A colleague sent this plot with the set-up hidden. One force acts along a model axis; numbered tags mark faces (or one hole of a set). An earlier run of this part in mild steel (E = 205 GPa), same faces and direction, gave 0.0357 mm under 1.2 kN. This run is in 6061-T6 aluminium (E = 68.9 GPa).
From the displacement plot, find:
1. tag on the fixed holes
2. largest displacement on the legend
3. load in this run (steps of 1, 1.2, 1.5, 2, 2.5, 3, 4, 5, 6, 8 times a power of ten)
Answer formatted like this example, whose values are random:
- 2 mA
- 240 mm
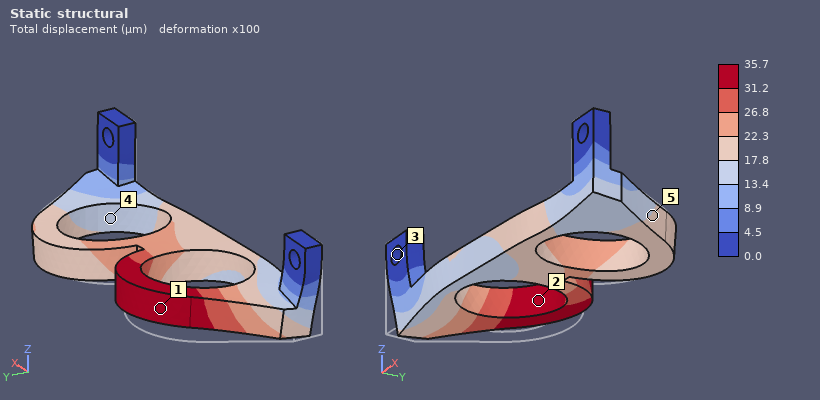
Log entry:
- 3
- 35.7 µm
- 400 N
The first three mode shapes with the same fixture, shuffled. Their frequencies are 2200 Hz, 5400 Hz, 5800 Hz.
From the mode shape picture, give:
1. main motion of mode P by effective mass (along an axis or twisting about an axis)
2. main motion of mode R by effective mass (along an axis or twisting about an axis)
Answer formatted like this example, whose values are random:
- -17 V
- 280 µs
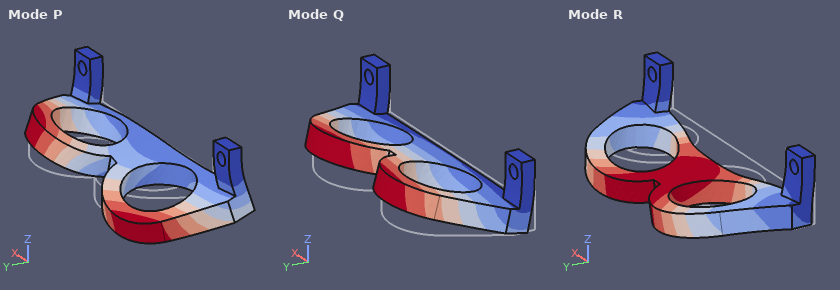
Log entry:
- along X
- along Y
